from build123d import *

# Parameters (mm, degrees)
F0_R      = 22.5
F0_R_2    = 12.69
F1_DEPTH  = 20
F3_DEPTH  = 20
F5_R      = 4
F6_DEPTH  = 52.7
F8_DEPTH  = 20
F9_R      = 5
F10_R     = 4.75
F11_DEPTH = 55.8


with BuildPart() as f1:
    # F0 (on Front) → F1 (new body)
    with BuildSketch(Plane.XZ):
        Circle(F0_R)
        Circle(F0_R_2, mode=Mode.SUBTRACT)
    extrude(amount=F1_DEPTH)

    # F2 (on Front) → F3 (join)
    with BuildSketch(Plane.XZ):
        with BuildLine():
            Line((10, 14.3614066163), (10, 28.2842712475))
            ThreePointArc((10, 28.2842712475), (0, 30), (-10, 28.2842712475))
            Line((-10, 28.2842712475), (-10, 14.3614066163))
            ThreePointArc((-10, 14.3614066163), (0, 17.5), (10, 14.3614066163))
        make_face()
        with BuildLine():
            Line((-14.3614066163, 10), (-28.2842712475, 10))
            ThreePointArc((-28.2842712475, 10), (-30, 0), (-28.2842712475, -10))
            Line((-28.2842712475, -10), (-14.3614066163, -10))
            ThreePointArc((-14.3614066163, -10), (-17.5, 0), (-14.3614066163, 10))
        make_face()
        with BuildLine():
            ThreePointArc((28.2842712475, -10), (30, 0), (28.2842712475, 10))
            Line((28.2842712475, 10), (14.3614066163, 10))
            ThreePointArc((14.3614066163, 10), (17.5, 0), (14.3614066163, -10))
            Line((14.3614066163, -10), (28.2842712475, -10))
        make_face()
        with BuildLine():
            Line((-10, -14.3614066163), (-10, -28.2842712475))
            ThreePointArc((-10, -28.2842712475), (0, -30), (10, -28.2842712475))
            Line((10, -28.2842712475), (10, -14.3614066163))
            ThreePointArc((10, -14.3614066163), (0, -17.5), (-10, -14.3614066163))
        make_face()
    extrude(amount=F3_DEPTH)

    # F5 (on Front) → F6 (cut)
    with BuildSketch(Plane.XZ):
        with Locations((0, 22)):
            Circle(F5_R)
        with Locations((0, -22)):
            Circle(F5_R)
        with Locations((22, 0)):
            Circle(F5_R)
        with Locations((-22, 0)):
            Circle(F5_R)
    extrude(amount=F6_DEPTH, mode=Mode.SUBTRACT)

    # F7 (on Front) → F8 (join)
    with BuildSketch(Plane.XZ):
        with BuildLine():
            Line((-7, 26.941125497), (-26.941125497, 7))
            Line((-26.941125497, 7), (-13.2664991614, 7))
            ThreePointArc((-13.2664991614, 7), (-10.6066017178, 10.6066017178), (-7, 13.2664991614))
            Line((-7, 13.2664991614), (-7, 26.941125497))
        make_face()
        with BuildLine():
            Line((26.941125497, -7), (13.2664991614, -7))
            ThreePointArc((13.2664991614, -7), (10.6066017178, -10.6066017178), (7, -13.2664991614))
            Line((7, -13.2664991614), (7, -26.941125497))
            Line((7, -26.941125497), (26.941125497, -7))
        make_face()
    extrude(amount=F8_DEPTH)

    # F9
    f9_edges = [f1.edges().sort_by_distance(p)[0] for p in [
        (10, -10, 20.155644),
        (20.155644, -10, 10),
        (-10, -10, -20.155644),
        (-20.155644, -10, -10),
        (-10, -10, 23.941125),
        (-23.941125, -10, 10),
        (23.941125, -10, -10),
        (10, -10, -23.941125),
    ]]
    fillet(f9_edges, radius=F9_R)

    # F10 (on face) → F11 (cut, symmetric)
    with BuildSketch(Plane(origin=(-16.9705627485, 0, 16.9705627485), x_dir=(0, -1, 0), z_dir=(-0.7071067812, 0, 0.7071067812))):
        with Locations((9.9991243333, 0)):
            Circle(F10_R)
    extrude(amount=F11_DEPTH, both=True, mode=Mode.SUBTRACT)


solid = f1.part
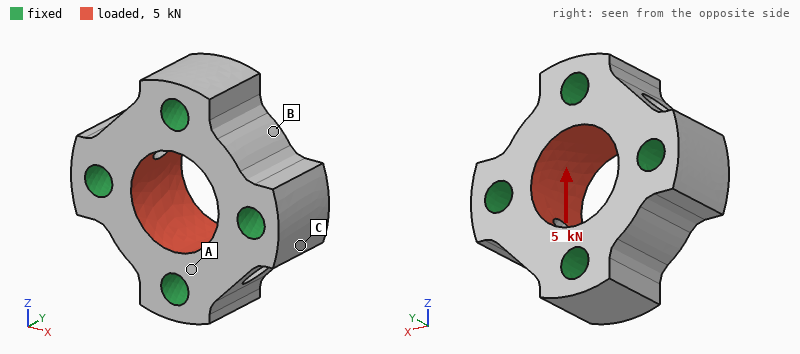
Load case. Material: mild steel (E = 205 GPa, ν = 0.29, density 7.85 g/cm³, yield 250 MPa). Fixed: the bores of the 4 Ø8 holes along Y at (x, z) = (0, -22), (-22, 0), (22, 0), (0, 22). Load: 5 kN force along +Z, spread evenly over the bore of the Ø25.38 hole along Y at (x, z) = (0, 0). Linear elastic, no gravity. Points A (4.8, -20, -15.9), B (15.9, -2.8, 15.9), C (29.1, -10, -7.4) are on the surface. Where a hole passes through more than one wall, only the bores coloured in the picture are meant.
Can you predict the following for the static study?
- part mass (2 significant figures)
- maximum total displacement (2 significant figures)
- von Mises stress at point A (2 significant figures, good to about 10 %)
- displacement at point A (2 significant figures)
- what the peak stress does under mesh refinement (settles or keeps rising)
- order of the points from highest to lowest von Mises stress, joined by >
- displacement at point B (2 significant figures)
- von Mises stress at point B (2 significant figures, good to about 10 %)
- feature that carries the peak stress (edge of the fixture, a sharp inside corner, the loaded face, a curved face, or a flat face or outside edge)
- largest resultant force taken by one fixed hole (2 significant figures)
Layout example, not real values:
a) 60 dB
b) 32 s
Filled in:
a) 230 g
b) 0.42 µm
c) 5.1 MPa
d) 0.13 µm
e) keeps rising
f) A > B > C
g) 0.30 µm
h) 3.3 MPa
i) edge of the fixture
j) 1.4 kN
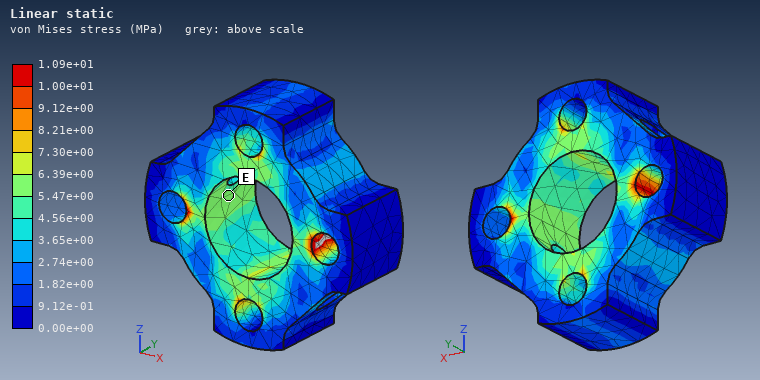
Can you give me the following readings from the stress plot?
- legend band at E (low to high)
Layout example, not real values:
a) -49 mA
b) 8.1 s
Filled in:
a) 5.47e+00 to 6.39e+00 MPa
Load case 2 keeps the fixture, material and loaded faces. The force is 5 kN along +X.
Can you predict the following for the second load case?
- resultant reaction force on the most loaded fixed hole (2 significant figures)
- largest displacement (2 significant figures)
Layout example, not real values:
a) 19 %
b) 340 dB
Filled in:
a) 1.4 kN
b) 0.42 µm
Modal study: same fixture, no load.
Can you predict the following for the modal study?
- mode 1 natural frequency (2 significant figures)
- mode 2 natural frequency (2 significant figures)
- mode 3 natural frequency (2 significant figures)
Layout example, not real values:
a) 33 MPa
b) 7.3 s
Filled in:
a) 48 kHz
b) 54 kHz
c) 56 kHz
